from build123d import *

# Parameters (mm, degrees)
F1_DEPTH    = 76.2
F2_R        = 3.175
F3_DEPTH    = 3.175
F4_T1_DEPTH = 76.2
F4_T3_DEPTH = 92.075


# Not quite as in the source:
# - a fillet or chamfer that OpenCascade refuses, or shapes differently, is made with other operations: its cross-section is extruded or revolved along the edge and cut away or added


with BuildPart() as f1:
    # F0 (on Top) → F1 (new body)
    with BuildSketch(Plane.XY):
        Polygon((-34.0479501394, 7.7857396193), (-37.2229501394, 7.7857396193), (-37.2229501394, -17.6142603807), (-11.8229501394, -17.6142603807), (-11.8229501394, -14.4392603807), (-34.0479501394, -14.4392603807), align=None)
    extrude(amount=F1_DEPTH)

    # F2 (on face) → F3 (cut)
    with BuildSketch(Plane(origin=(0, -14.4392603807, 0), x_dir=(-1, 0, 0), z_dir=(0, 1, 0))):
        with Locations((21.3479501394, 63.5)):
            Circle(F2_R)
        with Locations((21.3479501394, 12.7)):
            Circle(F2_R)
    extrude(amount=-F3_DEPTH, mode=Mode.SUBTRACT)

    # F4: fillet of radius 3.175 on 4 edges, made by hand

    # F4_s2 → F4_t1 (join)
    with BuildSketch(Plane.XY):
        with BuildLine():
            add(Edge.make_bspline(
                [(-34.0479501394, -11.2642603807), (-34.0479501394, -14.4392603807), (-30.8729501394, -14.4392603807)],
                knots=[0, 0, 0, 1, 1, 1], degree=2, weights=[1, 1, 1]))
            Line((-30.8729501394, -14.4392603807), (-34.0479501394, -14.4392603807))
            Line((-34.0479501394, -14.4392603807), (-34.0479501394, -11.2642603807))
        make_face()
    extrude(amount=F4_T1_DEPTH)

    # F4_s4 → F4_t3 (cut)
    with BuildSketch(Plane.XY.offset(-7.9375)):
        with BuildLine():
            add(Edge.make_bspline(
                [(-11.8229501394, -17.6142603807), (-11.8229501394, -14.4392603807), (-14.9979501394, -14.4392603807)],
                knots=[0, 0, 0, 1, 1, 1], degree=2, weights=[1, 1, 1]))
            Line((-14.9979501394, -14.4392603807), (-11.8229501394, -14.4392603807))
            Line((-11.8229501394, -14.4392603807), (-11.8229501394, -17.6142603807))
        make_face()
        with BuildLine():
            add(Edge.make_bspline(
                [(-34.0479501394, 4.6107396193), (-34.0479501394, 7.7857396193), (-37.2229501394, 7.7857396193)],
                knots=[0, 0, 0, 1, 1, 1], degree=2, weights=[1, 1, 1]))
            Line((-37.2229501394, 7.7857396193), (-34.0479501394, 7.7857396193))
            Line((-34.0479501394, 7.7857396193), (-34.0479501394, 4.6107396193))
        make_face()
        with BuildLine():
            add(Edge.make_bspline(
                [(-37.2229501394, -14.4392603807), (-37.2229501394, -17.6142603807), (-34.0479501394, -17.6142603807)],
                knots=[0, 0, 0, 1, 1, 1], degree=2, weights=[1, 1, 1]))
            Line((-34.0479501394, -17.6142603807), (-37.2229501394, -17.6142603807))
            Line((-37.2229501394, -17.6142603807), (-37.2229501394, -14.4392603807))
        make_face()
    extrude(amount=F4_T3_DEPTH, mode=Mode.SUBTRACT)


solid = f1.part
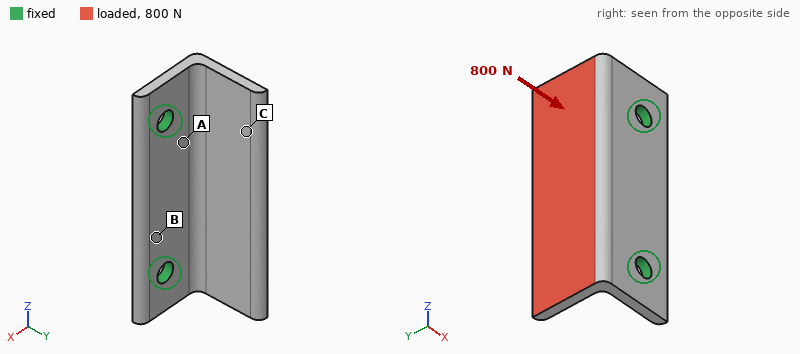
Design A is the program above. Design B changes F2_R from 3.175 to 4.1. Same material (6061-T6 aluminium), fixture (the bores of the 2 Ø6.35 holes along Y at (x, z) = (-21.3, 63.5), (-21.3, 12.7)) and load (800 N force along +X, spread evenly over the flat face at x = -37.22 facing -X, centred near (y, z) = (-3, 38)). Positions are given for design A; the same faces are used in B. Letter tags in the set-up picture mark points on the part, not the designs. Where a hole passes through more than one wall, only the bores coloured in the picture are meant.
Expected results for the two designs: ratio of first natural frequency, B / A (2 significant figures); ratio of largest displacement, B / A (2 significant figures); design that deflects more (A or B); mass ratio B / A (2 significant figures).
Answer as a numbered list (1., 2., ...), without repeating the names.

1. 1.1
2. 0.90
3. A
4. 0.99
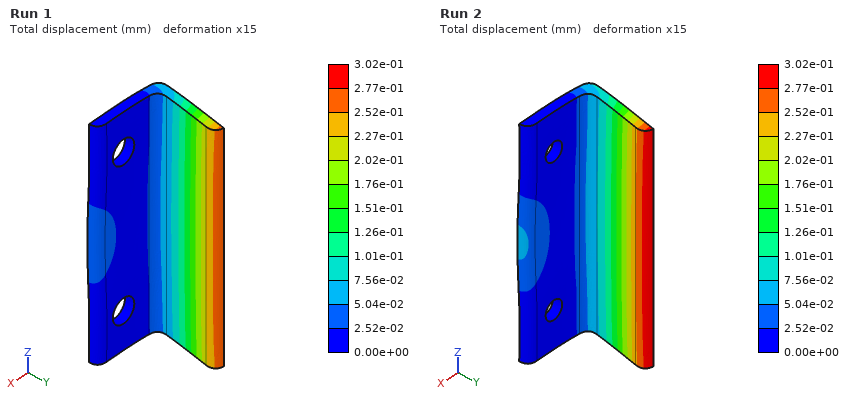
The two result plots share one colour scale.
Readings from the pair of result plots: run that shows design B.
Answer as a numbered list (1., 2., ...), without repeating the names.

1. Run 1
